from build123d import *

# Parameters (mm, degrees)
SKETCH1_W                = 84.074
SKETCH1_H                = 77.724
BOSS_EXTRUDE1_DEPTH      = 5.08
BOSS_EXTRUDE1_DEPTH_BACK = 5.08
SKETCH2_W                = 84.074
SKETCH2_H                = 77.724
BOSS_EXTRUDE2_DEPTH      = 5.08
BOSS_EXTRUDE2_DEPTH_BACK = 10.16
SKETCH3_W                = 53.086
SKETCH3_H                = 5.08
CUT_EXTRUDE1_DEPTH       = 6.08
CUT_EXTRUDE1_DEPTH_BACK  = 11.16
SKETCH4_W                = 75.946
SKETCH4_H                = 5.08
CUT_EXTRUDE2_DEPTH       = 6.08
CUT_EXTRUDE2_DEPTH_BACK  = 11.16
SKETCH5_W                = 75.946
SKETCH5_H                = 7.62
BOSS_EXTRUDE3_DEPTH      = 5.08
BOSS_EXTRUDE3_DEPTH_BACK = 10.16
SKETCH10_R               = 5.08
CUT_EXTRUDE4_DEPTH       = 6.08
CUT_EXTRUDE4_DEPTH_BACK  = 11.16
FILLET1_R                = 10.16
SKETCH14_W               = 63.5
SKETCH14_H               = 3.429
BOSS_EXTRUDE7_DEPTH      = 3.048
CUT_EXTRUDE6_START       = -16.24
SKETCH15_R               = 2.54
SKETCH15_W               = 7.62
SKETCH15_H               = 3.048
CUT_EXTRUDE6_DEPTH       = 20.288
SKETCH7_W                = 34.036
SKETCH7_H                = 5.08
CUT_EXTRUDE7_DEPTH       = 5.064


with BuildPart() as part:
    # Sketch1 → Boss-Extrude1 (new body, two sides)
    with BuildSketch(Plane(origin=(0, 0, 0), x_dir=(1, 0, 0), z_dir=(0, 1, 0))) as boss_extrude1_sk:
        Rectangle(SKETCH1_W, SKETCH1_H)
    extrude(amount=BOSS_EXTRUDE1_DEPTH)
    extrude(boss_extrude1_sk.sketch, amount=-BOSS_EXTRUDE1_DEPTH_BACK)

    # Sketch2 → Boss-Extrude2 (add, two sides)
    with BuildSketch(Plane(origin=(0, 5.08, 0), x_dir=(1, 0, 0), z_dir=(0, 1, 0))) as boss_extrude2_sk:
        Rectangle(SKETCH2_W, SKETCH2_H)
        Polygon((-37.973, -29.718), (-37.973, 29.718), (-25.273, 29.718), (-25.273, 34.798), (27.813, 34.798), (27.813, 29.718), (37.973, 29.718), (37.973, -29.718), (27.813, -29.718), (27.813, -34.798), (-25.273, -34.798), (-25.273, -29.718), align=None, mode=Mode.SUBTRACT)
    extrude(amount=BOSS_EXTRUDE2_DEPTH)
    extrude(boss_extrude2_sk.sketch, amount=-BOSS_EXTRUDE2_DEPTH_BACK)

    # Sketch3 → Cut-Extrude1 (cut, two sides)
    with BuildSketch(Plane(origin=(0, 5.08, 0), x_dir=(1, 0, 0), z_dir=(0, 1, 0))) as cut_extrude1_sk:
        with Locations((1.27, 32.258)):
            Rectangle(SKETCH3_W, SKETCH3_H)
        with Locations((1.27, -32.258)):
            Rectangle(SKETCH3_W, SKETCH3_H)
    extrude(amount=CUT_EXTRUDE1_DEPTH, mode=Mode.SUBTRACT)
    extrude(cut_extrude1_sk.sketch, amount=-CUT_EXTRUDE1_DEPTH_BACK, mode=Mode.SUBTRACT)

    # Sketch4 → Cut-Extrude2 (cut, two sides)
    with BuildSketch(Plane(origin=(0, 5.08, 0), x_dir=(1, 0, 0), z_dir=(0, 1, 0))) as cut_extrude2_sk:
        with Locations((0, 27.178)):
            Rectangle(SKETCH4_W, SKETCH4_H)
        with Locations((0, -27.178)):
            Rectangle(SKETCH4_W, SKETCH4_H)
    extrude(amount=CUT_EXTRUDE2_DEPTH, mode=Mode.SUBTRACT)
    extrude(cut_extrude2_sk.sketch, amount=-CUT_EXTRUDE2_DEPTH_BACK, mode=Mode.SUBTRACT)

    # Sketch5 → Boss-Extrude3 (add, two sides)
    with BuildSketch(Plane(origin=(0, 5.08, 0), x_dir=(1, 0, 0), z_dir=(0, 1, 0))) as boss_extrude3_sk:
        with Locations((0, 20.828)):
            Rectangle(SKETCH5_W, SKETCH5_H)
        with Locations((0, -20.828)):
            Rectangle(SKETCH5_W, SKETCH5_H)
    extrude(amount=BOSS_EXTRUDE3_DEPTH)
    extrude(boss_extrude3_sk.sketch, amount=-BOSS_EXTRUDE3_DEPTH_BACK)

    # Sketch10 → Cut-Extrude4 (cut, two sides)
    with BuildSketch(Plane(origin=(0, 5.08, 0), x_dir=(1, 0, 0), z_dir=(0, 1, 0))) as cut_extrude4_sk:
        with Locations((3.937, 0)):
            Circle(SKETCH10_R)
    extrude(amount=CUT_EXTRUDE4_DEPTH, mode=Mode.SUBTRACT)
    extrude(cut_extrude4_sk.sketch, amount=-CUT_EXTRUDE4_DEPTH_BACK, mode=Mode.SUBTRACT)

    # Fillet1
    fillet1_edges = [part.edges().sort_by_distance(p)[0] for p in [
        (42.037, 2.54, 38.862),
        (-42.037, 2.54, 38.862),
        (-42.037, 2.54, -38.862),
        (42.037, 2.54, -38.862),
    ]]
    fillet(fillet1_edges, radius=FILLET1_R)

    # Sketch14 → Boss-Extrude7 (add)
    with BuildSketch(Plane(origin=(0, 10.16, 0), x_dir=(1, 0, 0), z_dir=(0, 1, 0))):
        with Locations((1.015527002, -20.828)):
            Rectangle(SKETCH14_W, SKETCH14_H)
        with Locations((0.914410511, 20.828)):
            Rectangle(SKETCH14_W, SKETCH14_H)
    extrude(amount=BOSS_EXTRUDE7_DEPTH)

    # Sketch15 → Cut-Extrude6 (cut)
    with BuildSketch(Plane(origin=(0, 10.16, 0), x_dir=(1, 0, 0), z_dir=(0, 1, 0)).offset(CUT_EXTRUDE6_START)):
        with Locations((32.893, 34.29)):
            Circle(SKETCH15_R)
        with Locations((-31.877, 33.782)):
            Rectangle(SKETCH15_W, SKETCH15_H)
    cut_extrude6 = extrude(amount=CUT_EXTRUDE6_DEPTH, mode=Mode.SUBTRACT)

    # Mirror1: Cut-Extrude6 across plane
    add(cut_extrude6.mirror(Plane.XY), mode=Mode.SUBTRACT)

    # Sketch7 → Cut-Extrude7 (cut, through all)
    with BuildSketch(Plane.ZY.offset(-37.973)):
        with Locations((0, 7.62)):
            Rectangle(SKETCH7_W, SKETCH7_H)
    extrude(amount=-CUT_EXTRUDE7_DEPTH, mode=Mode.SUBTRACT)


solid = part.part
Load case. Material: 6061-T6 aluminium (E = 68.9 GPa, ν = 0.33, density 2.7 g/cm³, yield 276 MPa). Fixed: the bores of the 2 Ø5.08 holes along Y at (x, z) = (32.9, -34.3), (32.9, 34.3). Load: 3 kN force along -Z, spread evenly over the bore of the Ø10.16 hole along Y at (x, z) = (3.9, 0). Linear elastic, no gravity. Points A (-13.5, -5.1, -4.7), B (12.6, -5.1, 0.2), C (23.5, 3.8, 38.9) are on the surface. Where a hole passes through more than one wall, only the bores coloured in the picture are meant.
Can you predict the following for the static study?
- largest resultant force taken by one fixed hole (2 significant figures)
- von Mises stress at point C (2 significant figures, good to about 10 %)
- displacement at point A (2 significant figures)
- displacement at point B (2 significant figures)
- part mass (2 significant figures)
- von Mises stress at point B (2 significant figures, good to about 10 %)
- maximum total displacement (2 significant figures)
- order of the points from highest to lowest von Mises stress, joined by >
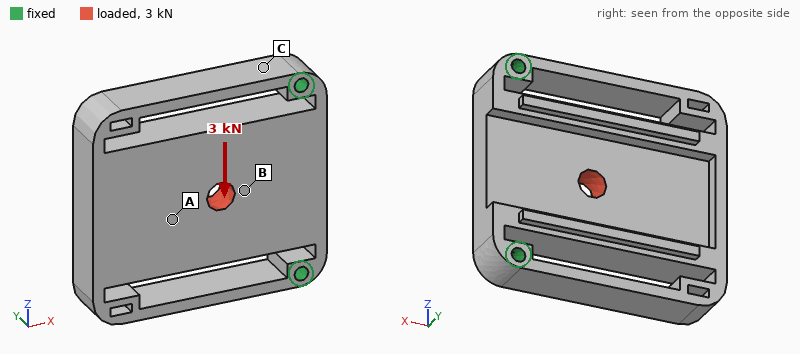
2.3 kN
33 MPa
0.082 mm
0.049 mm
170 g
18 MPa
0.13 mm
C > B > A
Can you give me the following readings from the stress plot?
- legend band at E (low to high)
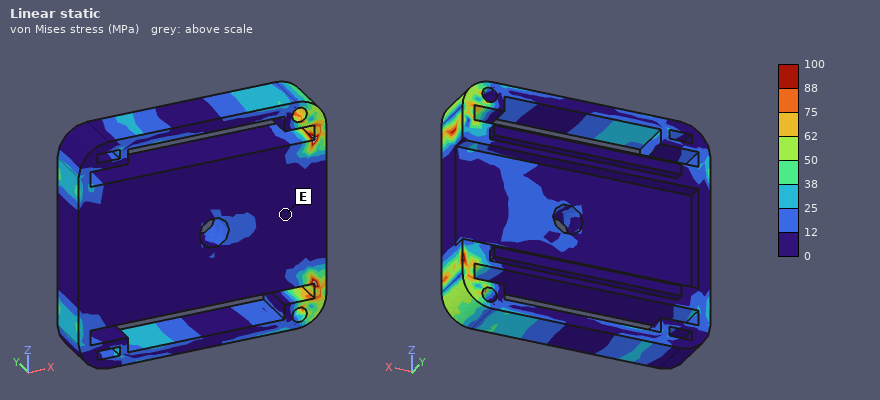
0 to 12 MPa
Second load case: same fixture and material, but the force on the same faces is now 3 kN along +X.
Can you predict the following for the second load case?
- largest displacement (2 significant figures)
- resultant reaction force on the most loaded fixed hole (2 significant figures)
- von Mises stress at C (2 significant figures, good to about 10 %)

64 µm
1.5 kN
13 MPa
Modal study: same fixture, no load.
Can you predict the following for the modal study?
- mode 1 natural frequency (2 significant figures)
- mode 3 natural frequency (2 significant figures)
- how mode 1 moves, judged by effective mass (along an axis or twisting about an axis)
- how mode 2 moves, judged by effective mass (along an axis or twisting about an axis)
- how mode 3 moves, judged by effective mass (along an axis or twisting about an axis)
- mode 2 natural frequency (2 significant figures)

900 Hz
2800 Hz
along Y
along Z
twisting about X
2000 Hz
